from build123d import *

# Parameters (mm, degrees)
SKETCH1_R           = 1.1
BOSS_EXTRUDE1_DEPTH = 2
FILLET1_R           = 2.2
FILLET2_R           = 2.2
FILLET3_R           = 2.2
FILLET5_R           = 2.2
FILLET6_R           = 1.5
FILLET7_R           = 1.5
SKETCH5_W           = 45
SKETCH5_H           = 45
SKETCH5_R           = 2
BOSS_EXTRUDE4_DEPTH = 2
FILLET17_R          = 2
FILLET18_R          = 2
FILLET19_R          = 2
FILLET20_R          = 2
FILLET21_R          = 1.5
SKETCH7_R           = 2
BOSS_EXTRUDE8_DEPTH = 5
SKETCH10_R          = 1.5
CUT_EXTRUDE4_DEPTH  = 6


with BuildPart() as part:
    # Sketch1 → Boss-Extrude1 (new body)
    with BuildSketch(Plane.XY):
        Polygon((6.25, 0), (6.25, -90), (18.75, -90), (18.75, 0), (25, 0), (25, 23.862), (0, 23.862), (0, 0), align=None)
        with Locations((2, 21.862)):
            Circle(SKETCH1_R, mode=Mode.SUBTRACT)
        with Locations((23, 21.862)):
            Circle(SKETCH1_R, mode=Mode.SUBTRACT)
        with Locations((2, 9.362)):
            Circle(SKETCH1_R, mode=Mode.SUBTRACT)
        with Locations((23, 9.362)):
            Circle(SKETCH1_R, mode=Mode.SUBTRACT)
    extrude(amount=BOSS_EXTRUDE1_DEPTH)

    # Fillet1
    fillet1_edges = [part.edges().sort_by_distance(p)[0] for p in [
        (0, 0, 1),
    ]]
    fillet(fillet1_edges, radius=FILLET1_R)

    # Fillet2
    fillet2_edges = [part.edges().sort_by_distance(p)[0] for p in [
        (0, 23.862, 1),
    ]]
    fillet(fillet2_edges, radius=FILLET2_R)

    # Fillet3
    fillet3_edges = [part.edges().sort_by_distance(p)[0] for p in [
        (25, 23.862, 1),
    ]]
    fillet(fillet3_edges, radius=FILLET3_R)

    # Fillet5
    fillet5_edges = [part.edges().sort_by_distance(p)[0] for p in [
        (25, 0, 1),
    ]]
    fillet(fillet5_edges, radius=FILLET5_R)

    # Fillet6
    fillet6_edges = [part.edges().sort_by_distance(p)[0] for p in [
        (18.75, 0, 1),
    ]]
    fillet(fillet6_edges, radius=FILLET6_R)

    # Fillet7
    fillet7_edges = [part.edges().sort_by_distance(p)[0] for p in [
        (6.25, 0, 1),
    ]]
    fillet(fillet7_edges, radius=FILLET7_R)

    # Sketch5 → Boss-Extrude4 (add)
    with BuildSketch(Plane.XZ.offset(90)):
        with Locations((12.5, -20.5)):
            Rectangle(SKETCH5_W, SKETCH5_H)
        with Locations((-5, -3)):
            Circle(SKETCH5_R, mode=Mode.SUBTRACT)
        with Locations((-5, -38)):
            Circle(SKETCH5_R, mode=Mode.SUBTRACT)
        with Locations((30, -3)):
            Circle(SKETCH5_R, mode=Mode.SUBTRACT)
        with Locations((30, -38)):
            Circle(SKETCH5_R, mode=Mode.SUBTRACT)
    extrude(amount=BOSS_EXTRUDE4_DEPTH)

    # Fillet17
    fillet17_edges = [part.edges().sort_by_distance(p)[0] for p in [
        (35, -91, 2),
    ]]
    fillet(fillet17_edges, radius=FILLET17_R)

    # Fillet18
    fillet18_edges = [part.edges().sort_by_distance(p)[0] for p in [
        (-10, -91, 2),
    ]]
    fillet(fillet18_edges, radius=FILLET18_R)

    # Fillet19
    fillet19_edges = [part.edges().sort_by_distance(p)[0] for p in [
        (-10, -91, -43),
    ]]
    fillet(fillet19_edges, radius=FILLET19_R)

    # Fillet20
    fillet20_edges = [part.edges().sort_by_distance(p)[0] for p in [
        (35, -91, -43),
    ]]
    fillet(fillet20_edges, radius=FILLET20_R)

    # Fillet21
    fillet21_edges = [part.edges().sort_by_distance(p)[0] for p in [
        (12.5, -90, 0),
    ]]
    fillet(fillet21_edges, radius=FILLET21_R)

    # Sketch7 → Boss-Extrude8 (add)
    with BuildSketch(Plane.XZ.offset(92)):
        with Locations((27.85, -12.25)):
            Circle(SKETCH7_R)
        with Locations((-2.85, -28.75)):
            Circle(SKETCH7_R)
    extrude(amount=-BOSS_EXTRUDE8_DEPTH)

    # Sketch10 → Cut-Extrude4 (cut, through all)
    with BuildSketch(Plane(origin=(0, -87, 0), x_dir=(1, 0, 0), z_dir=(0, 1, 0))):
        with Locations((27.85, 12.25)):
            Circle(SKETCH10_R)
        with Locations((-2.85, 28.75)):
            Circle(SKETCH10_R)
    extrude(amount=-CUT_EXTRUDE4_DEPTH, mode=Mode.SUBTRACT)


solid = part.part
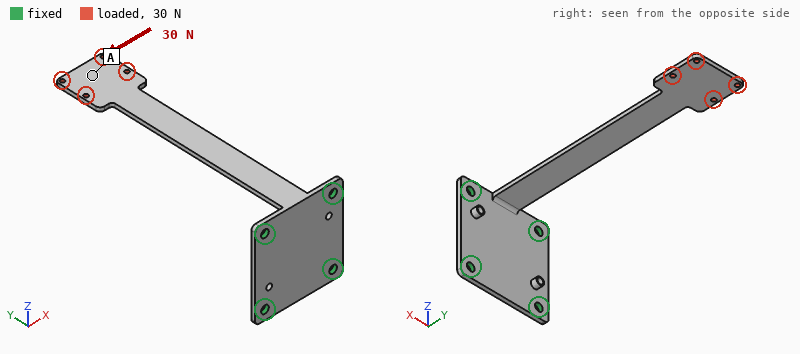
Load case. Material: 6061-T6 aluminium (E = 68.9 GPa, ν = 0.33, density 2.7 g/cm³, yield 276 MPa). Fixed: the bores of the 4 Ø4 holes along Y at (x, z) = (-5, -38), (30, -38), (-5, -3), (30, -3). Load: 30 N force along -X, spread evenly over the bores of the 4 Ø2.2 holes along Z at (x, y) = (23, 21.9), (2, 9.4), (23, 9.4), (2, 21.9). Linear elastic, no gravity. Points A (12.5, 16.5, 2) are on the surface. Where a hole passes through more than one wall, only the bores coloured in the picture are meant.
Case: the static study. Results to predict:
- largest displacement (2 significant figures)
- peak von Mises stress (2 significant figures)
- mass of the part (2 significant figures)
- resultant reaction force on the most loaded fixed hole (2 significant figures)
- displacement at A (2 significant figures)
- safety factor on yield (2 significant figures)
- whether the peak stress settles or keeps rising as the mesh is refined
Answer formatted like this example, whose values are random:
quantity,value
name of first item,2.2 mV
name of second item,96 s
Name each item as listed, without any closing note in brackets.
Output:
quantity,value
largest displacement,1.3 mm
peak von Mises stress,270 MPa
mass of the part,20 g
resultant reaction force on the most loaded fixed hole,140 N
displacement at A,1.2 mm
safety factor on yield,1.0
whether the peak stress settles or keeps rising as the mesh is refined,settles
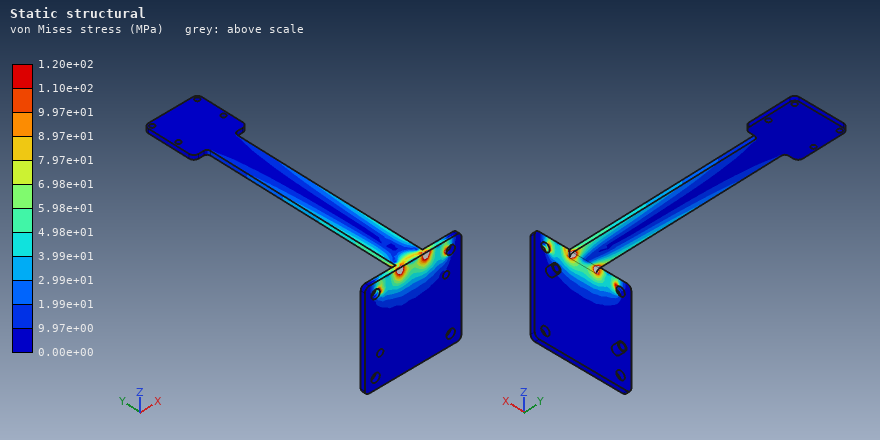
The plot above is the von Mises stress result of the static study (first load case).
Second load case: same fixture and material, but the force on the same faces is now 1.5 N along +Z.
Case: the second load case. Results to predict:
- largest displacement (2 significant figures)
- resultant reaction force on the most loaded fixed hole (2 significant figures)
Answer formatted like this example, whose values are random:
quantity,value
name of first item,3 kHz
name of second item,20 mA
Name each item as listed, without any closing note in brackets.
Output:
quantity,value
largest displacement,1.3 mm
resultant reaction force on the most loaded fixed hole,3.0 N
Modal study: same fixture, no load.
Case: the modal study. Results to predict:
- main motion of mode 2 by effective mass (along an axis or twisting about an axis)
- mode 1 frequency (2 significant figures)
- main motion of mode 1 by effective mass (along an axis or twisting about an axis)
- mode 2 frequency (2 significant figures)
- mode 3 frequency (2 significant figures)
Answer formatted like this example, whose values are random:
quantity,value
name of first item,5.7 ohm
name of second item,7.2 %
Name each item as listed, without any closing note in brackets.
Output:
quantity,value
main motion of mode 2 by effective mass,along X
mode 1 frequency,95 Hz
main motion of mode 1 by effective mass,along Z
mode 2 frequency,400 Hz
mode 3 frequency,690 Hz
